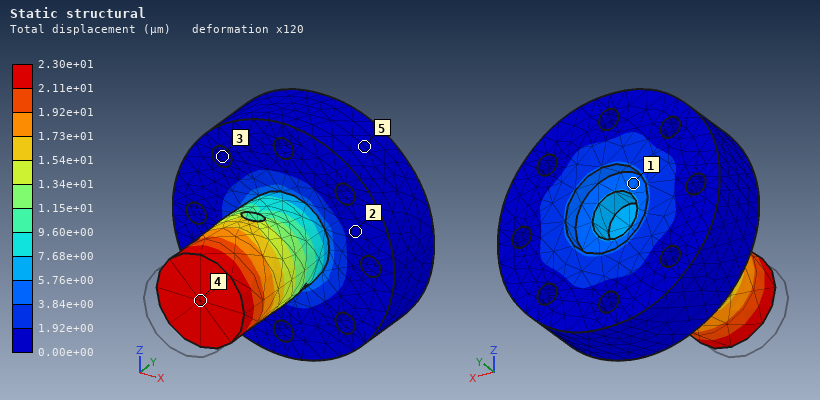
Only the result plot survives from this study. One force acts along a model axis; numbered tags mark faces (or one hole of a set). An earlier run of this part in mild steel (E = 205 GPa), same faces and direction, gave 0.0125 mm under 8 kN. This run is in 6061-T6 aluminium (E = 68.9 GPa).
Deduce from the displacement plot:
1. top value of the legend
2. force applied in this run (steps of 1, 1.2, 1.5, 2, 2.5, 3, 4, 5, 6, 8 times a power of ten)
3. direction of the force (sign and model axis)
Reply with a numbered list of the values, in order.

1. 2.30e+01 µm
2. 5 kN
3. +Y
